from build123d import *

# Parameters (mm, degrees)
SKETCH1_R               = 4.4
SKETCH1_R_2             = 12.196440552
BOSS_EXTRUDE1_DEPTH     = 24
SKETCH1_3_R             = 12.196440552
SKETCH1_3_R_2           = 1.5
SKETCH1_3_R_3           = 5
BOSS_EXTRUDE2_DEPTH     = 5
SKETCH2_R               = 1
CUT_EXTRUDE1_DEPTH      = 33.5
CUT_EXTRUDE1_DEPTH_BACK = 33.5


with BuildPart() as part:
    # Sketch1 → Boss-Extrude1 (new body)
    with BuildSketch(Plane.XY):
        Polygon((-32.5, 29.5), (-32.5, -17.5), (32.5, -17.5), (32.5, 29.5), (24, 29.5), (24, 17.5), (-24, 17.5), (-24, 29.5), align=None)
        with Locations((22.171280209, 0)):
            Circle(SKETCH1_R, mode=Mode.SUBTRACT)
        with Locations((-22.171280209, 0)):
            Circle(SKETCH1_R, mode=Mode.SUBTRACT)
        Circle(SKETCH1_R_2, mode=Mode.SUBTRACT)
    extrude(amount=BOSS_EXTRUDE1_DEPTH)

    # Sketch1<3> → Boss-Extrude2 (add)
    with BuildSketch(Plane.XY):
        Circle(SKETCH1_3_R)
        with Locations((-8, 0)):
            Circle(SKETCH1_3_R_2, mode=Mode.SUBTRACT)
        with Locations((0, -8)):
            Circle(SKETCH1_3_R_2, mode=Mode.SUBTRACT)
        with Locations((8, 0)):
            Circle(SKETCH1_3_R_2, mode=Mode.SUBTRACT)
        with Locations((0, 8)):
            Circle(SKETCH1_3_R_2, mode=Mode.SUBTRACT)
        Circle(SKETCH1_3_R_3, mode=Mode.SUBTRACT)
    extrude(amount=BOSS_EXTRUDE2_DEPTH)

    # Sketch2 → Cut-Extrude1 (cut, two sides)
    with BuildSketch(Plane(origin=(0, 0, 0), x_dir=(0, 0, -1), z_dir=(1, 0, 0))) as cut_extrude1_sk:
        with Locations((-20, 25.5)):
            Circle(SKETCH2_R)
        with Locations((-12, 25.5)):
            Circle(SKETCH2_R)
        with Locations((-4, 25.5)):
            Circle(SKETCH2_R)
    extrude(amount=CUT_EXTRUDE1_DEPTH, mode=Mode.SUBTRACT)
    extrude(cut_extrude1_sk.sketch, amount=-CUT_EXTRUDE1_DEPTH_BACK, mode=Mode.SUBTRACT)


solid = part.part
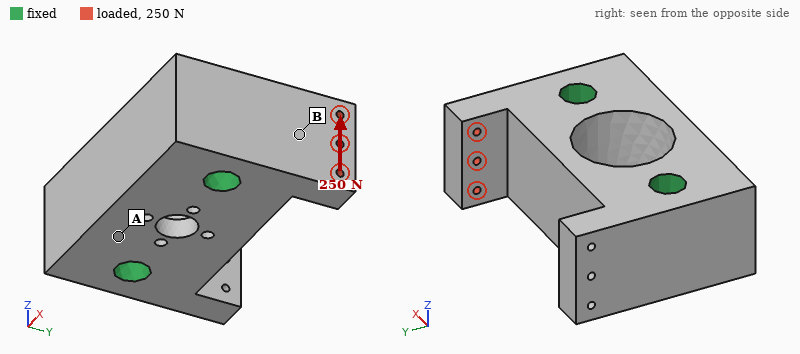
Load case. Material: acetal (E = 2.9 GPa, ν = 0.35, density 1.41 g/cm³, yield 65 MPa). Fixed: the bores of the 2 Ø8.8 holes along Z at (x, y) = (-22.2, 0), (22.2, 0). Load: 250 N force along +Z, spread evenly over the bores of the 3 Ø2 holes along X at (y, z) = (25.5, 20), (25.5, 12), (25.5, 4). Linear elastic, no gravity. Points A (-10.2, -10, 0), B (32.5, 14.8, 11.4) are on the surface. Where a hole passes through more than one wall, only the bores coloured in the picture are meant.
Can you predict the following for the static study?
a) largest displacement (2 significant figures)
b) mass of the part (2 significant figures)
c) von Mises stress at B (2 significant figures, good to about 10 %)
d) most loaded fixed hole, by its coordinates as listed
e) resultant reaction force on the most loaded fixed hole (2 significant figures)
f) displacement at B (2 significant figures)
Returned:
58 µm
66 g
2.1 MPa
(22.2, 0)
250 N
17 µm
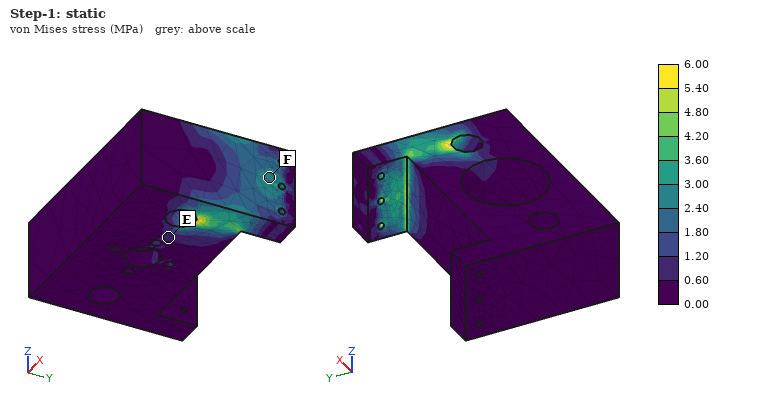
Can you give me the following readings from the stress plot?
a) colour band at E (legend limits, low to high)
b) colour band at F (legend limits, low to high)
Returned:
0.60 to 1.20 MPa
2.40 to 3.00 MPa
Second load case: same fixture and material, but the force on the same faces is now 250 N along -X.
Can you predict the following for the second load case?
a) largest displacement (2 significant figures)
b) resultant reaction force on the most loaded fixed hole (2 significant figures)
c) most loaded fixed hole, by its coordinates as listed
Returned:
0.11 mm
170 N
(22.2, 0)
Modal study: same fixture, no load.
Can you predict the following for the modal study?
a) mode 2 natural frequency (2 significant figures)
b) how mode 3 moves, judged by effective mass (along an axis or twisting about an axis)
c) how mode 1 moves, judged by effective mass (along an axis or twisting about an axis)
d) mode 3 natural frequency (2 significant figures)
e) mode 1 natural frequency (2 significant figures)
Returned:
5400 Hz
along Z
along X
6200 Hz
5000 Hz
